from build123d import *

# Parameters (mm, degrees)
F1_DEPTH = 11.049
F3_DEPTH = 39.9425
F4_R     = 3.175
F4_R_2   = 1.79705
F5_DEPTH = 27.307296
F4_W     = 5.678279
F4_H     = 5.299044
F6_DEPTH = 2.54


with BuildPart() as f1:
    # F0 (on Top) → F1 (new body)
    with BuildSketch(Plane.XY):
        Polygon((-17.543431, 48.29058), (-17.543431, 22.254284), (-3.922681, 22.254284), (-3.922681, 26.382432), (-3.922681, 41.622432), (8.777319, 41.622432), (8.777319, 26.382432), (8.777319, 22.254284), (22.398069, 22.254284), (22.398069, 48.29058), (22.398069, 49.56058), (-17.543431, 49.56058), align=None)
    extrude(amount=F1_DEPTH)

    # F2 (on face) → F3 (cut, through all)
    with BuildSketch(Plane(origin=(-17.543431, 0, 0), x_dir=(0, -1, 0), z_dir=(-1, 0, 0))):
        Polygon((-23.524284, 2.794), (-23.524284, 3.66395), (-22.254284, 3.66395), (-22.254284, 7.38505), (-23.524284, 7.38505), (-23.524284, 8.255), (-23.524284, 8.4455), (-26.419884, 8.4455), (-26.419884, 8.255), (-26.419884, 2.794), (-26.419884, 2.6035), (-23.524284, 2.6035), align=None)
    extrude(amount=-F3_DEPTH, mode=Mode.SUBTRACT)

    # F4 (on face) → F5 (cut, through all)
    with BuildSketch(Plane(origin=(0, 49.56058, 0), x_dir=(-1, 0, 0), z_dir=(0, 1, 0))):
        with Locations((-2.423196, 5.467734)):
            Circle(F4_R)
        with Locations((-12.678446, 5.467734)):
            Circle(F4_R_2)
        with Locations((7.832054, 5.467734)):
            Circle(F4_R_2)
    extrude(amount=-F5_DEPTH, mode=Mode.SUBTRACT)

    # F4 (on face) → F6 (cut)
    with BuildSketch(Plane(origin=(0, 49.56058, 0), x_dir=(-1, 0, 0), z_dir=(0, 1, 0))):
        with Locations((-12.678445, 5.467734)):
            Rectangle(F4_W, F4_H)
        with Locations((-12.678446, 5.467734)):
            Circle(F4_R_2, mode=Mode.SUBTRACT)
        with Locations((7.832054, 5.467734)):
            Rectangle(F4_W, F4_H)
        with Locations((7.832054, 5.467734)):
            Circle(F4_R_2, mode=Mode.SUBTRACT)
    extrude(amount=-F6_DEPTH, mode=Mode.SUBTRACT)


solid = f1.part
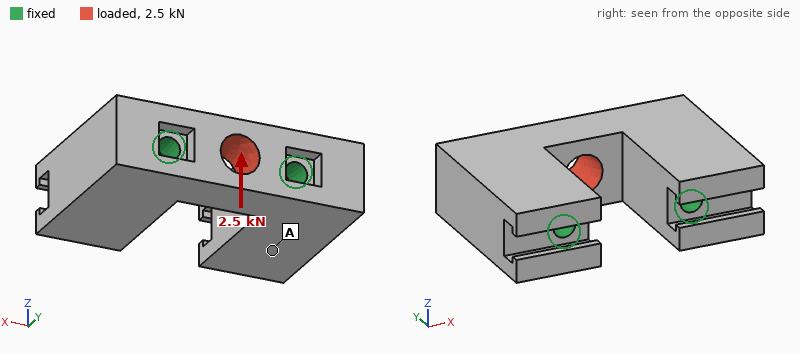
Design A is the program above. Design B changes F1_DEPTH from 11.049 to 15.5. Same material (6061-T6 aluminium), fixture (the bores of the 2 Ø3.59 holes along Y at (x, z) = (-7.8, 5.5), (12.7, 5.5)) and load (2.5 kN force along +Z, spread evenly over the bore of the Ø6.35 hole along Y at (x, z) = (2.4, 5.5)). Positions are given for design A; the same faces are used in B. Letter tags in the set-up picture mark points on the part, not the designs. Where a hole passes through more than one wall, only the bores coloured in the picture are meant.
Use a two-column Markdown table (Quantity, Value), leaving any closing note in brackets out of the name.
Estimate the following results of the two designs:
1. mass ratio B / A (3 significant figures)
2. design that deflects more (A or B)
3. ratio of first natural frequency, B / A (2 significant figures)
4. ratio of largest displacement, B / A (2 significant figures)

| Quantity | Value |
|---|---|
| mass ratio B / A | 1.47 |
| design that deflects more | A |
| ratio of first natural frequency, B / A | 0.77 |
| ratio of largest displacement, B / A | 0.81 |
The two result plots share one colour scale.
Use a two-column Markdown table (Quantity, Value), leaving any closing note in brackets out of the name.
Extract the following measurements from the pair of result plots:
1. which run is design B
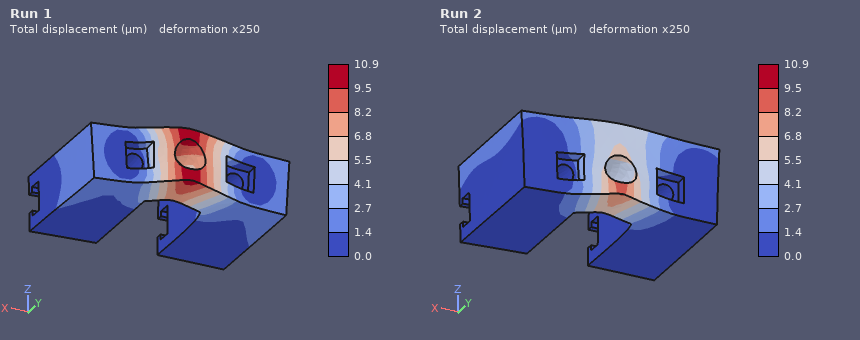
| Quantity | Value |
|---|---|
| which run is design B | Run 2 |
